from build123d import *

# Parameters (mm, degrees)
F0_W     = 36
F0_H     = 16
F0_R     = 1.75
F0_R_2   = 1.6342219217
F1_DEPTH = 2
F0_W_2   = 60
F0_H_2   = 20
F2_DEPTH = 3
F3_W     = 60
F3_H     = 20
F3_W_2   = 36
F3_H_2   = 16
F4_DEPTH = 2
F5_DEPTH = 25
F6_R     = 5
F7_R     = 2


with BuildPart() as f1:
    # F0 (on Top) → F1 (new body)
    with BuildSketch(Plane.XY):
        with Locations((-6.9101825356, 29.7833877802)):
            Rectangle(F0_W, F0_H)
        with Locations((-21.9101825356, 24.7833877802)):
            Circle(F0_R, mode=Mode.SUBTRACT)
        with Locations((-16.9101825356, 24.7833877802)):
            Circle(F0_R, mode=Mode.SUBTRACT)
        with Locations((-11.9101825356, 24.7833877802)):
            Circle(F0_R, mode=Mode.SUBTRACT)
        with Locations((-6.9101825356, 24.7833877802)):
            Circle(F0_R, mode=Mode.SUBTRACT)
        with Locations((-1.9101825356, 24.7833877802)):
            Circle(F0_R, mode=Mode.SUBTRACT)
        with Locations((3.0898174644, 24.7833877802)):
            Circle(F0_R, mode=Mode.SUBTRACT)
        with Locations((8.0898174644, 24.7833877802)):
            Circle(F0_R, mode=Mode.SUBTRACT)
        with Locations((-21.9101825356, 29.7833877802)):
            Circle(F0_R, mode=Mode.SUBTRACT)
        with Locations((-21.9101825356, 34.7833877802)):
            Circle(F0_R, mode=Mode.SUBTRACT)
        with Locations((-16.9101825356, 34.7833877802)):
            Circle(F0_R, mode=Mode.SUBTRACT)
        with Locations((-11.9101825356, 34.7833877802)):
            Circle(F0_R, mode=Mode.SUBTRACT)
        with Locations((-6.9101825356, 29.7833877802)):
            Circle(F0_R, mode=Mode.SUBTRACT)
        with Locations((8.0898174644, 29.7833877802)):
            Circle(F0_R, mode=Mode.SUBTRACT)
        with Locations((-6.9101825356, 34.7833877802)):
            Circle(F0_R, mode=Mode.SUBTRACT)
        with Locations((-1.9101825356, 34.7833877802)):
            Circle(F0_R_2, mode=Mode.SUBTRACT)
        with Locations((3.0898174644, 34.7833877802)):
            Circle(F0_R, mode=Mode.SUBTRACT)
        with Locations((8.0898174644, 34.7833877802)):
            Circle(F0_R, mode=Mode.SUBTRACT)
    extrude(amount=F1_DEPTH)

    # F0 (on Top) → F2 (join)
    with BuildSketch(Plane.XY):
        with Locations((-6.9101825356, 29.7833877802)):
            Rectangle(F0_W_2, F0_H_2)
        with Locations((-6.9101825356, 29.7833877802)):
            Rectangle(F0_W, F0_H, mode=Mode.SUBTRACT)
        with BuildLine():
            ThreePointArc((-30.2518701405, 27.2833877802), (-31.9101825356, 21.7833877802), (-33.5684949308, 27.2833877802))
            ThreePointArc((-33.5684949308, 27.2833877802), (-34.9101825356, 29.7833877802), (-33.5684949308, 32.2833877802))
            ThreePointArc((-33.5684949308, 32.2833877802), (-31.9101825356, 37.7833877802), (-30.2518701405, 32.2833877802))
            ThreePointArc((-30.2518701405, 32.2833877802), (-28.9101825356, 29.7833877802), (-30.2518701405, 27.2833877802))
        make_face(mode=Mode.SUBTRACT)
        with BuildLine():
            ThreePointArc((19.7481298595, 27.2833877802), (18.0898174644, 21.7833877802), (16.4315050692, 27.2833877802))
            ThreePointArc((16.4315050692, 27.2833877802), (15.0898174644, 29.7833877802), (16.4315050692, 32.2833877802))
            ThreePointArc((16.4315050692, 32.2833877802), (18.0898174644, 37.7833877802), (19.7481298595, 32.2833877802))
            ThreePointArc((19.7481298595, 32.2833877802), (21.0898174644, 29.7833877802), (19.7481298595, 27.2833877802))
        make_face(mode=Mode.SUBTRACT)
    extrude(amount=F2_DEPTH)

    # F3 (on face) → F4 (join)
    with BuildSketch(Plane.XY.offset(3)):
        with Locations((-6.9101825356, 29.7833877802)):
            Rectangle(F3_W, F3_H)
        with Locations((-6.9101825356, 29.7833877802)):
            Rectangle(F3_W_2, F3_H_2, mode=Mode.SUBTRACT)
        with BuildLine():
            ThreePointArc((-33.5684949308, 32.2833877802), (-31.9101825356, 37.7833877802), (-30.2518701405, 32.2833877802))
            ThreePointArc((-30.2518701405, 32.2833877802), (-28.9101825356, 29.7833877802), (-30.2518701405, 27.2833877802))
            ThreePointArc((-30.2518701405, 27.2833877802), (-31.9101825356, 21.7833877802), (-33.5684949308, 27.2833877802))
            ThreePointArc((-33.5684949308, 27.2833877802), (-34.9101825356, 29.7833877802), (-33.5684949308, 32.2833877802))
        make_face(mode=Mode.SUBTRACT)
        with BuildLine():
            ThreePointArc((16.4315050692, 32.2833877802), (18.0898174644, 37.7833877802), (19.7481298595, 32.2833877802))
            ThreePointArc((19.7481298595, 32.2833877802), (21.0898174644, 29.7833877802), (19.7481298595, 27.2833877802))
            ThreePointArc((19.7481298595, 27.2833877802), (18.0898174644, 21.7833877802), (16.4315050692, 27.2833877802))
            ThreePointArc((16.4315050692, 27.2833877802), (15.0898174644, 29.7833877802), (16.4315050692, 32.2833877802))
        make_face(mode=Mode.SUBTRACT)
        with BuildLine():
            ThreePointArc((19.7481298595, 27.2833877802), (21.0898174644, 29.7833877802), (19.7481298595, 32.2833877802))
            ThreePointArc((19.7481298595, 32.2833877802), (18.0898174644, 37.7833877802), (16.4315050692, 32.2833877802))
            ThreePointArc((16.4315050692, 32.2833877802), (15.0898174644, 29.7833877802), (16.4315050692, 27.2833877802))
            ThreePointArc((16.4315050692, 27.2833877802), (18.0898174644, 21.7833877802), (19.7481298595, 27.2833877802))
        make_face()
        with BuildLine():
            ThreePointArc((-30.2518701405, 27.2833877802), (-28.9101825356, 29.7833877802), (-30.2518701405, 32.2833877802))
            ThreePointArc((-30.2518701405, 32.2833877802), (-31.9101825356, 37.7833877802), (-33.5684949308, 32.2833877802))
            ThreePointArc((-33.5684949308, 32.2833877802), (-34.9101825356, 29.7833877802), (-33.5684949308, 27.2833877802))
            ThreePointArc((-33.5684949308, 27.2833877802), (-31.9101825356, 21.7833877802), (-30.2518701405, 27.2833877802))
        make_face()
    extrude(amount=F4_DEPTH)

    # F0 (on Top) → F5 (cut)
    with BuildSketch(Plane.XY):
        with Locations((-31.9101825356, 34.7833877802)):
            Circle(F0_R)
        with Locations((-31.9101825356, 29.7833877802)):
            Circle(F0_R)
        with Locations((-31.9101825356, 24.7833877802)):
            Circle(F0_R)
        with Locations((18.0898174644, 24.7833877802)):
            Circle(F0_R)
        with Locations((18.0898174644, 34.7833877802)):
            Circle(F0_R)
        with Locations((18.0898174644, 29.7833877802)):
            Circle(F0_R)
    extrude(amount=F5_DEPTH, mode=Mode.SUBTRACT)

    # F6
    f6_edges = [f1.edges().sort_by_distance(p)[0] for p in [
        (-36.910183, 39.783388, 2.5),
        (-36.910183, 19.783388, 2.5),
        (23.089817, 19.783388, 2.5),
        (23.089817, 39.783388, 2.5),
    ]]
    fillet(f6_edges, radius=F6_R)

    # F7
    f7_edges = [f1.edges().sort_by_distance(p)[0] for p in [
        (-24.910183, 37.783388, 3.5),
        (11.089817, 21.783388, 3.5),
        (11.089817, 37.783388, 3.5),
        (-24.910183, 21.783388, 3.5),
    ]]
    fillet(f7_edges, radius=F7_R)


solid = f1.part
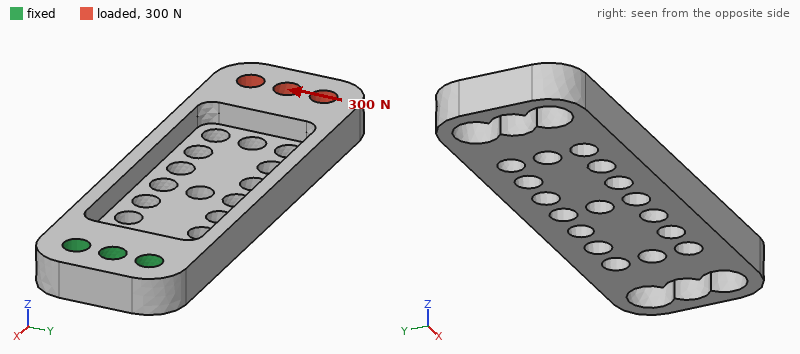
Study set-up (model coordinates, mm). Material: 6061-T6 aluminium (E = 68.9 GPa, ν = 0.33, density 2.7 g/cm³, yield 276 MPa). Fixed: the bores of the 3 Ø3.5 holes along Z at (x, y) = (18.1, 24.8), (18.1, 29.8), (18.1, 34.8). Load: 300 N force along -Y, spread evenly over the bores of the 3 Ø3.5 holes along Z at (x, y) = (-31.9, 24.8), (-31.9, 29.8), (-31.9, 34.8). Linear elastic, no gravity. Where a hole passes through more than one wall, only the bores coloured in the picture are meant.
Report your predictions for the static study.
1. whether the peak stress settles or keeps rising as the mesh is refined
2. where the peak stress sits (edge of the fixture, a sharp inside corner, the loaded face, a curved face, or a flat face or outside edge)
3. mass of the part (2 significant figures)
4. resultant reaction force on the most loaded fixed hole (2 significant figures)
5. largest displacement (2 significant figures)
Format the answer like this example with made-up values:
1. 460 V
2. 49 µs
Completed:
1. keeps rising
2. edge of the fixture
3. 8.8 g
4. 1.1 kN
5. 0.34 mm
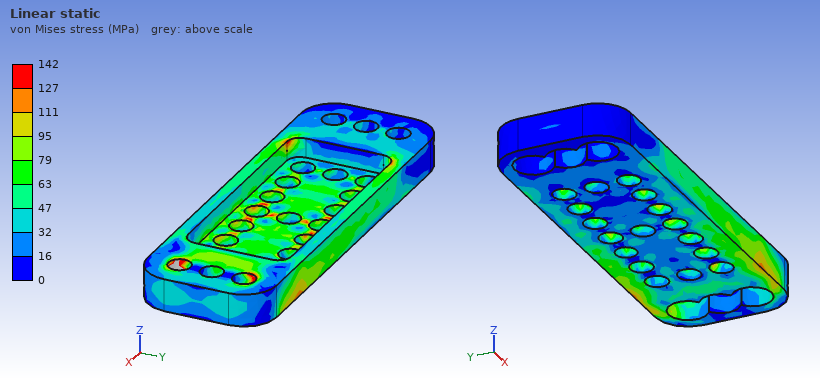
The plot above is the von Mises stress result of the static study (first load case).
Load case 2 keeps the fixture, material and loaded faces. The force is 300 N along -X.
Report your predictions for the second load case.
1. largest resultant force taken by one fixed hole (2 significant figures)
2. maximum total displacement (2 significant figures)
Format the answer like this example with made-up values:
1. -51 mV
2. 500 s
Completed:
1. 140 N
2. 0.18 mm
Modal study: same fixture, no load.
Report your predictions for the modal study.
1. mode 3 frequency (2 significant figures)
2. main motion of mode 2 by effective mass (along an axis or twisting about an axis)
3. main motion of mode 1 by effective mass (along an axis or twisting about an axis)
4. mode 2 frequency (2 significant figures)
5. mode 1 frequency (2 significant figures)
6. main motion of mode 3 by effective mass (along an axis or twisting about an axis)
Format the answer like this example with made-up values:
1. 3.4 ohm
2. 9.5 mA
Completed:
1. 4600 Hz
2. along Y
3. along Z
4. 2700 Hz
5. 960 Hz
6. along Y
